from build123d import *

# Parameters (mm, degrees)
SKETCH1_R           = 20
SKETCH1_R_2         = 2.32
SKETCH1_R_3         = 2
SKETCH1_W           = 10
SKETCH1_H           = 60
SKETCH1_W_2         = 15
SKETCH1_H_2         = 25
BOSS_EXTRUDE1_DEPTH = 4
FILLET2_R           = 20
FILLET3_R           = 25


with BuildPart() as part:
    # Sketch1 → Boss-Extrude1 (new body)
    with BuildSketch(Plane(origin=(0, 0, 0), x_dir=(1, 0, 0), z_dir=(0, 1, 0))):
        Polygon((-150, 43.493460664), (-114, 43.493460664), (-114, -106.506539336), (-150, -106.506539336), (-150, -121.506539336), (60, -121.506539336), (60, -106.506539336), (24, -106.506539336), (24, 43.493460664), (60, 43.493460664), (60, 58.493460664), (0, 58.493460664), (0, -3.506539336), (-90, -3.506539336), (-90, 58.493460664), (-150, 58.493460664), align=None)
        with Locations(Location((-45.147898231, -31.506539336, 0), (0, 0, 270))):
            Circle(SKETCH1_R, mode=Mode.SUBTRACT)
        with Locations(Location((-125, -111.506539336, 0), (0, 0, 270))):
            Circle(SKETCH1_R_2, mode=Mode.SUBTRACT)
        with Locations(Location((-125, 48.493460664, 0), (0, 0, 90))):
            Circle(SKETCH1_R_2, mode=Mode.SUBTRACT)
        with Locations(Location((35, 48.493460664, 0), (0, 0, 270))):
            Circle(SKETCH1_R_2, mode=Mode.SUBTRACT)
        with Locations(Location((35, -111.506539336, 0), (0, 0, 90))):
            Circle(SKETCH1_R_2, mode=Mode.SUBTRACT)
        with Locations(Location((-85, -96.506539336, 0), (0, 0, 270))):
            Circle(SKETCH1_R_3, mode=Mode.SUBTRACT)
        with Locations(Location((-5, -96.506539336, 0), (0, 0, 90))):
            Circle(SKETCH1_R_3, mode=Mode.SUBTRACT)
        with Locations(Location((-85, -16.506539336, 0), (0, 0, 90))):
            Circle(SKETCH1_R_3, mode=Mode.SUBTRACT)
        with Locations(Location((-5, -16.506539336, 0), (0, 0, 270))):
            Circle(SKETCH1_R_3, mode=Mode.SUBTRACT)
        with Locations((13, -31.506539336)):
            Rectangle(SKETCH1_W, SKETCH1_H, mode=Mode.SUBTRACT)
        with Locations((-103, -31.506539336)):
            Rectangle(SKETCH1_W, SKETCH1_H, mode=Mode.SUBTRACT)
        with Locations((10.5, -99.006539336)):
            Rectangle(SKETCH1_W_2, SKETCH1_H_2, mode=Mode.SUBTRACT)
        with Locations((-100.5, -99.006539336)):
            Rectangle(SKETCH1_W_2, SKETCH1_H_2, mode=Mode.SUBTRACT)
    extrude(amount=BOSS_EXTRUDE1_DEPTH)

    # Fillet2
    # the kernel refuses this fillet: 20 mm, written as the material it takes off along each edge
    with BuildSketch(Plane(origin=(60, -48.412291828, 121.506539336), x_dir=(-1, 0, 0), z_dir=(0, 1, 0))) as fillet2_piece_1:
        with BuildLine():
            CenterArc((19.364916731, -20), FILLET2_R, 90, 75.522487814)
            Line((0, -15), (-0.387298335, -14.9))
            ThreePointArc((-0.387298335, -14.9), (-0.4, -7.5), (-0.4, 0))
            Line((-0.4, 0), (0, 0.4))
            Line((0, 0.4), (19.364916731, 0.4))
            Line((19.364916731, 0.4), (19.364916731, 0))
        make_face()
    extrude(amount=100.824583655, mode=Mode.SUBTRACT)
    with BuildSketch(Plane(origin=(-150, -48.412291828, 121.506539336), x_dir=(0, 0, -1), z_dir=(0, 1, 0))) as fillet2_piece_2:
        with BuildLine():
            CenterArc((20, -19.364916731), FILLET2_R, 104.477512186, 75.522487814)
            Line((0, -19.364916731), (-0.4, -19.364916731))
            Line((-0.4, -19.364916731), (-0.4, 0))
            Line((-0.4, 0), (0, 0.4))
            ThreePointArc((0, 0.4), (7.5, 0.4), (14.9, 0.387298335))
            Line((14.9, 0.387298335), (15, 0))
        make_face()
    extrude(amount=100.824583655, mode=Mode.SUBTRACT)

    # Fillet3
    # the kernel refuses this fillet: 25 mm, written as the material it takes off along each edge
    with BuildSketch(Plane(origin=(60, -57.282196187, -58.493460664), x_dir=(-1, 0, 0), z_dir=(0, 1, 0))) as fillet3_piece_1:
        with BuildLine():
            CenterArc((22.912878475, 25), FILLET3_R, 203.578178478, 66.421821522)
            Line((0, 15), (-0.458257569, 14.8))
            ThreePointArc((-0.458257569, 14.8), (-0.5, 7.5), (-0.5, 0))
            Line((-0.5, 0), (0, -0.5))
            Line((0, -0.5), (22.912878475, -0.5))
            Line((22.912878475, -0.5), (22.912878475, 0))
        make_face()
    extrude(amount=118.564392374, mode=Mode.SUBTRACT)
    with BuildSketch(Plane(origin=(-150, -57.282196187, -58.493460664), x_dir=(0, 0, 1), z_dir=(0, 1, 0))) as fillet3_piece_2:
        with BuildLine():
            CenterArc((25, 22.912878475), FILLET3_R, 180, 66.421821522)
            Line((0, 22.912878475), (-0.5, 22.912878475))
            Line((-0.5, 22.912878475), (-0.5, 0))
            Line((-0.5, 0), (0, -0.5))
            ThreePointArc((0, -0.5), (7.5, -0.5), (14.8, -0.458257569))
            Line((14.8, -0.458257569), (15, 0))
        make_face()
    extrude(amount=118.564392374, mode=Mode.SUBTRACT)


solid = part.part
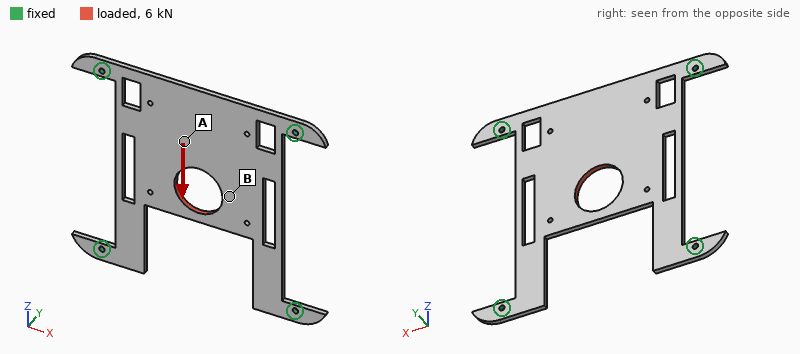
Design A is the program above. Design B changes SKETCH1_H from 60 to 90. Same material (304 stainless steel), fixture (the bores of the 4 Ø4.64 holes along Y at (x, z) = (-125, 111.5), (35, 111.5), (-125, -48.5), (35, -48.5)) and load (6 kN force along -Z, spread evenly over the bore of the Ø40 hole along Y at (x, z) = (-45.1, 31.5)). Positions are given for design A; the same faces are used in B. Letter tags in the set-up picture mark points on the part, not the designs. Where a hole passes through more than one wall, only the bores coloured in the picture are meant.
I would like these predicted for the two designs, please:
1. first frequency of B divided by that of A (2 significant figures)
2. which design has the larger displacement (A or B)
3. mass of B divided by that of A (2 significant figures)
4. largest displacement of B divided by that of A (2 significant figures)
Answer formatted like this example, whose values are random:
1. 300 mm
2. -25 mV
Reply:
1. 1.0
2. B
3. 0.97
4. 1.3
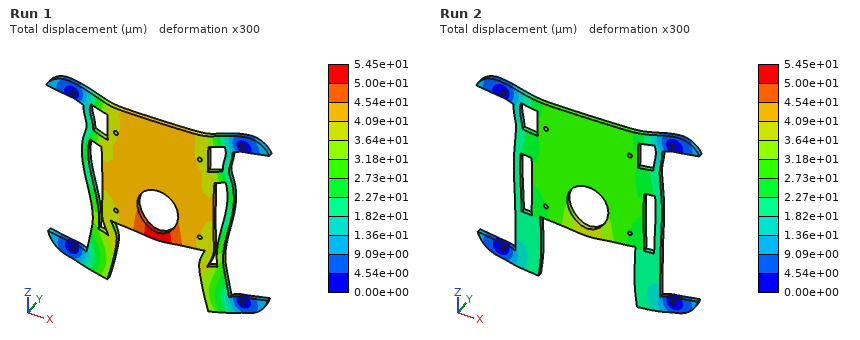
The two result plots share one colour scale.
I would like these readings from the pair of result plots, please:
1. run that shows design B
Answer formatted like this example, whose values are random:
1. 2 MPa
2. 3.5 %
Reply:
1. Run 1
